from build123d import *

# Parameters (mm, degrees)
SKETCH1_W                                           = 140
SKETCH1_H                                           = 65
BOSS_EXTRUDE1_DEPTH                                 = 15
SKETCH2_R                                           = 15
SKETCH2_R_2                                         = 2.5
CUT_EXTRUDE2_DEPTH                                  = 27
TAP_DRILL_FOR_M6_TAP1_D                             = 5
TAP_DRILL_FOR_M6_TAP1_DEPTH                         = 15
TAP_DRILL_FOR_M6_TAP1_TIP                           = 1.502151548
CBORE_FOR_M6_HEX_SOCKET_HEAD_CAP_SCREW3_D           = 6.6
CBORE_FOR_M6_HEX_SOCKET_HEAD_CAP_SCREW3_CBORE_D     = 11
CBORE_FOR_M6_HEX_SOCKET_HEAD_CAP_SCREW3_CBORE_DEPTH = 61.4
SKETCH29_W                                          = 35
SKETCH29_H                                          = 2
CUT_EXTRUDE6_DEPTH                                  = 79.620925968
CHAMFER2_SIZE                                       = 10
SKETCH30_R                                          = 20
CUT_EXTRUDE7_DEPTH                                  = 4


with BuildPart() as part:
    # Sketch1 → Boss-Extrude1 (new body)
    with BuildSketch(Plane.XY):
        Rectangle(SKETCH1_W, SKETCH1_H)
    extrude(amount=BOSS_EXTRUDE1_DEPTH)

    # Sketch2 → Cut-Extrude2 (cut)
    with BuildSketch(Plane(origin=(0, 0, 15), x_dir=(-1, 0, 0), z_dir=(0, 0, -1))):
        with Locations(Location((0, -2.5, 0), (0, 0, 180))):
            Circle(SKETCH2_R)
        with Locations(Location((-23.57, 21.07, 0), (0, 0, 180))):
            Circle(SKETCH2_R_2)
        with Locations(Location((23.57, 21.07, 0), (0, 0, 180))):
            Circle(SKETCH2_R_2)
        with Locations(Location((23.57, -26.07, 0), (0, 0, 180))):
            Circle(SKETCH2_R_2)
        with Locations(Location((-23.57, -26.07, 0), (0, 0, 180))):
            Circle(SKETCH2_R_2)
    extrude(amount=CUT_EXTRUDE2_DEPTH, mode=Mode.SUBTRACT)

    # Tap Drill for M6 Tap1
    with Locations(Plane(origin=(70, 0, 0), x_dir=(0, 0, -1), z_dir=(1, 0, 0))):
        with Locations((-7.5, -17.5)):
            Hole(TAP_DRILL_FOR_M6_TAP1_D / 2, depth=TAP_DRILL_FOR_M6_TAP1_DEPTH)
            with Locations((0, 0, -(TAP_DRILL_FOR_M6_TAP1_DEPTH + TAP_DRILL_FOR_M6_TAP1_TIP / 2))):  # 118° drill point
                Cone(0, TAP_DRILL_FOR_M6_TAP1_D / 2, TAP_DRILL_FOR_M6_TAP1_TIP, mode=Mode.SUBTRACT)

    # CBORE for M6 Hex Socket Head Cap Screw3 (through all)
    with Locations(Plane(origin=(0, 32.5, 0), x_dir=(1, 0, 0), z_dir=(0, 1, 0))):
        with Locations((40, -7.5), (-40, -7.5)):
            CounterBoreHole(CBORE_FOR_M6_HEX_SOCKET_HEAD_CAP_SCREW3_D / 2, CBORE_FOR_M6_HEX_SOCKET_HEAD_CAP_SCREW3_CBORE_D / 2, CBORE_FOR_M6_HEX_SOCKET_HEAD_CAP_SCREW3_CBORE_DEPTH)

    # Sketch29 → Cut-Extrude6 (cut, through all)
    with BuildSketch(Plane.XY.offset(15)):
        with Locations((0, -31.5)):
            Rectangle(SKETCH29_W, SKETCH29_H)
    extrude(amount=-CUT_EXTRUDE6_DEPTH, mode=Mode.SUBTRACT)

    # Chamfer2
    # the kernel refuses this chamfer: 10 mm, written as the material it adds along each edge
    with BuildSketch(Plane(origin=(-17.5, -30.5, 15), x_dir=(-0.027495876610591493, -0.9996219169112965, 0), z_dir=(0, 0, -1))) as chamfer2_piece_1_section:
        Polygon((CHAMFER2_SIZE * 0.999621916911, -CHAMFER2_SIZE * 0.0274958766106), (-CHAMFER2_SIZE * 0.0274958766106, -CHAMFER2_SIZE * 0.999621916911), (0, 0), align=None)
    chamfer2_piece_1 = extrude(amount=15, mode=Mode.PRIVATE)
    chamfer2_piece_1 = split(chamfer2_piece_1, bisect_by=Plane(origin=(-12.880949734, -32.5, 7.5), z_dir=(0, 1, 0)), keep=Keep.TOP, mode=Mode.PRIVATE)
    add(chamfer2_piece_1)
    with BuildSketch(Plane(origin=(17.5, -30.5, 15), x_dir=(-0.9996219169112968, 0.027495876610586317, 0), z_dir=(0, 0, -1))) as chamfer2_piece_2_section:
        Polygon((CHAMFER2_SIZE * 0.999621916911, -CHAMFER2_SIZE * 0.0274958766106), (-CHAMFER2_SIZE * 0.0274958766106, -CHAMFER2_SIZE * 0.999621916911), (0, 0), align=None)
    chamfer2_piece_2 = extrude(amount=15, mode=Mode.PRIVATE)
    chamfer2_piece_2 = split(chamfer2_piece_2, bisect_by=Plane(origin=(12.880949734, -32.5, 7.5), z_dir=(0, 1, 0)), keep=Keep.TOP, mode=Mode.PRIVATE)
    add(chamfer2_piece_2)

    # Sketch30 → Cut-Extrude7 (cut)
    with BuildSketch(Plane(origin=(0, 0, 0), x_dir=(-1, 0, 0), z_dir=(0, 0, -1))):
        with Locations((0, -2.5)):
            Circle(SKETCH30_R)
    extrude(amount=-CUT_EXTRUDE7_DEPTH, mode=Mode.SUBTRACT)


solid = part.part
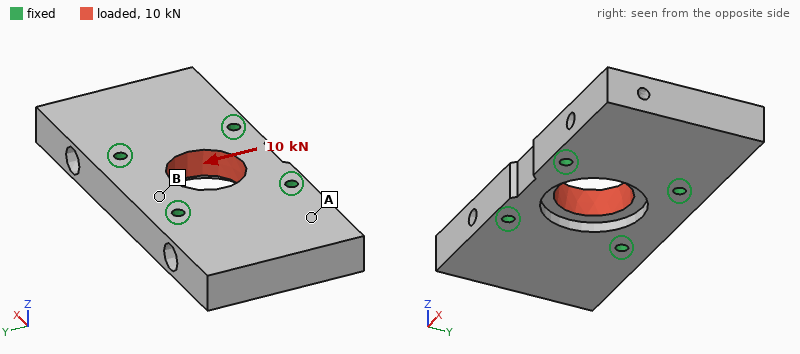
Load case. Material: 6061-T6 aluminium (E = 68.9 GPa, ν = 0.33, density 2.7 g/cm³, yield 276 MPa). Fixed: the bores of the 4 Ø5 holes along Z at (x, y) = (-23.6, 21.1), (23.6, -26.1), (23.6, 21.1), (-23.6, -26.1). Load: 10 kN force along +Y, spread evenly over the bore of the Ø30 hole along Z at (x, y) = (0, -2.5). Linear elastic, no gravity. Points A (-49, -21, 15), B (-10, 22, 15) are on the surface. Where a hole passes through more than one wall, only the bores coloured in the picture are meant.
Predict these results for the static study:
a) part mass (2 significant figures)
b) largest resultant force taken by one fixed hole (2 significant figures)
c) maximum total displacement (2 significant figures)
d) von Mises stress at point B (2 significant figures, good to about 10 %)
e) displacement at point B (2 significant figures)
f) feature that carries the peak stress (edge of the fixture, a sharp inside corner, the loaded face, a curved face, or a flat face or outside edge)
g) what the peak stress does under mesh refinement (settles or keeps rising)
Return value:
300 g
2.7 kN
8.6 µm
9.8 MPa
4.0 µm
edge of the fixture
keeps rising
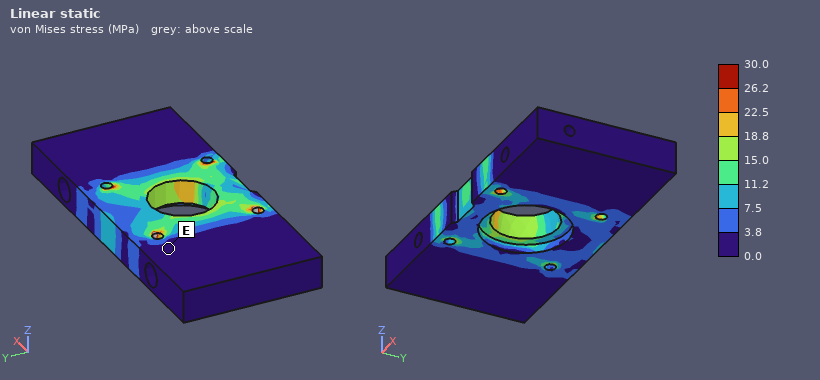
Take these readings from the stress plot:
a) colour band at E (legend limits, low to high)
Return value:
0.0 to 3.8 MPa
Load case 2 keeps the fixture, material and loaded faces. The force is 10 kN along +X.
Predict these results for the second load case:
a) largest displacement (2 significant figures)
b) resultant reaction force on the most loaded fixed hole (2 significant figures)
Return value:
5.5 µm
2.6 kN
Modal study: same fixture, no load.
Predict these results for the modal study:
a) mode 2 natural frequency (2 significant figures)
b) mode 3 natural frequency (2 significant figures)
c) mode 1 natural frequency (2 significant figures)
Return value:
3900 Hz
7500 Hz
3900 Hz
